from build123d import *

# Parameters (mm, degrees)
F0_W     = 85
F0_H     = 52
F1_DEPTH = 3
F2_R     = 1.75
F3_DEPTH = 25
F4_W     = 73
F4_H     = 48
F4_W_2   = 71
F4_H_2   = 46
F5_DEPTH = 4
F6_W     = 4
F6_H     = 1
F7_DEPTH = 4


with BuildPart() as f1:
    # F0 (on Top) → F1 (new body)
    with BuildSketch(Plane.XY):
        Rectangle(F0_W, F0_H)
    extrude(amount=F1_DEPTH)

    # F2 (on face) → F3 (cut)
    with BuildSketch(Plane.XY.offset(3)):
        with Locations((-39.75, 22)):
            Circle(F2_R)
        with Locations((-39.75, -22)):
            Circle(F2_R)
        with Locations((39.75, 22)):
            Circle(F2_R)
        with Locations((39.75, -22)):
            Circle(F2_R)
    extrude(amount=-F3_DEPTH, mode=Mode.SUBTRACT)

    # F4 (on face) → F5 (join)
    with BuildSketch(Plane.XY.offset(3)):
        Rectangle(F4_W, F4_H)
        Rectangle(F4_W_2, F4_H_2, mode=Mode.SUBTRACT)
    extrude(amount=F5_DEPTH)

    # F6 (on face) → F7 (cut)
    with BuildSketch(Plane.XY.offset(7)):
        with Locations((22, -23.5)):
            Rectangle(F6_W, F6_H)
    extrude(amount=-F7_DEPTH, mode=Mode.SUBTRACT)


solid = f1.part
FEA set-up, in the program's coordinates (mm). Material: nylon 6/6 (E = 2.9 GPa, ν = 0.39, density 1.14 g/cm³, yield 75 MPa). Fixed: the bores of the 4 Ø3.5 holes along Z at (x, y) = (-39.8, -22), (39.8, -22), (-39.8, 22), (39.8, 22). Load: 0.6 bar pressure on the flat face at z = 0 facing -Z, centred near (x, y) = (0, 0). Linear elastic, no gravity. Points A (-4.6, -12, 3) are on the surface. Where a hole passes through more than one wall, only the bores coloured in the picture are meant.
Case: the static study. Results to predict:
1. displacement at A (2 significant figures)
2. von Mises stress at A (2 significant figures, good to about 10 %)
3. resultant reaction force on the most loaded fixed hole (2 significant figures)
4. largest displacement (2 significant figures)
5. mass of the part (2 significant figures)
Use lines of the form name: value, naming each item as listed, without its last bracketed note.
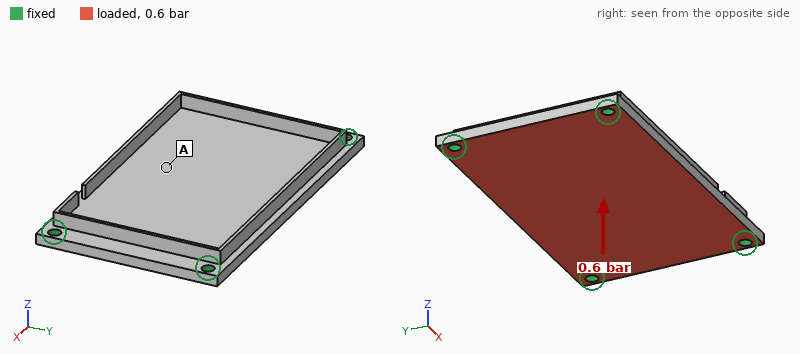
displacement at A: 0.89 mm
von Mises stress at A: 7.2 MPa
resultant reaction force on the most loaded fixed hole: 69 N
largest displacement: 0.95 mm
mass of the part: 16 g
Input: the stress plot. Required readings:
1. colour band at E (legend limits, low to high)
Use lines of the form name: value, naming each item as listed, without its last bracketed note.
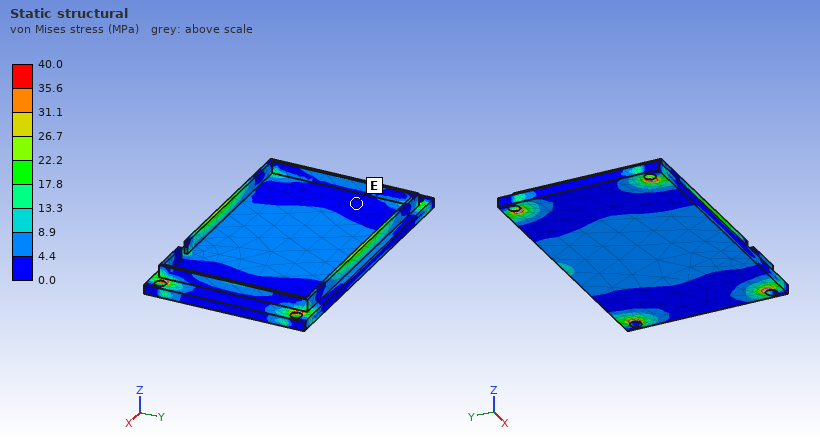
colour band at E: 0.0 to 4.4 MPa
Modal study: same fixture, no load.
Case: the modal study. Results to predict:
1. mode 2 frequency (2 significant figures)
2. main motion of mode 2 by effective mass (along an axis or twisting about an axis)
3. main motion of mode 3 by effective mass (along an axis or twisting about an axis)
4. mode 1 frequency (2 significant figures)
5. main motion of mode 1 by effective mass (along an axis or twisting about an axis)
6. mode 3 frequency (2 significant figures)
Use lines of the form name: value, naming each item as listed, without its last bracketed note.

mode 2 frequency: 1200 Hz
main motion of mode 2 by effective mass: twisting about X
main motion of mode 3 by effective mass: twisting about Y
mode 1 frequency: 770 Hz
main motion of mode 1 by effective mass: along Z
mode 3 frequency: 2000 Hz
